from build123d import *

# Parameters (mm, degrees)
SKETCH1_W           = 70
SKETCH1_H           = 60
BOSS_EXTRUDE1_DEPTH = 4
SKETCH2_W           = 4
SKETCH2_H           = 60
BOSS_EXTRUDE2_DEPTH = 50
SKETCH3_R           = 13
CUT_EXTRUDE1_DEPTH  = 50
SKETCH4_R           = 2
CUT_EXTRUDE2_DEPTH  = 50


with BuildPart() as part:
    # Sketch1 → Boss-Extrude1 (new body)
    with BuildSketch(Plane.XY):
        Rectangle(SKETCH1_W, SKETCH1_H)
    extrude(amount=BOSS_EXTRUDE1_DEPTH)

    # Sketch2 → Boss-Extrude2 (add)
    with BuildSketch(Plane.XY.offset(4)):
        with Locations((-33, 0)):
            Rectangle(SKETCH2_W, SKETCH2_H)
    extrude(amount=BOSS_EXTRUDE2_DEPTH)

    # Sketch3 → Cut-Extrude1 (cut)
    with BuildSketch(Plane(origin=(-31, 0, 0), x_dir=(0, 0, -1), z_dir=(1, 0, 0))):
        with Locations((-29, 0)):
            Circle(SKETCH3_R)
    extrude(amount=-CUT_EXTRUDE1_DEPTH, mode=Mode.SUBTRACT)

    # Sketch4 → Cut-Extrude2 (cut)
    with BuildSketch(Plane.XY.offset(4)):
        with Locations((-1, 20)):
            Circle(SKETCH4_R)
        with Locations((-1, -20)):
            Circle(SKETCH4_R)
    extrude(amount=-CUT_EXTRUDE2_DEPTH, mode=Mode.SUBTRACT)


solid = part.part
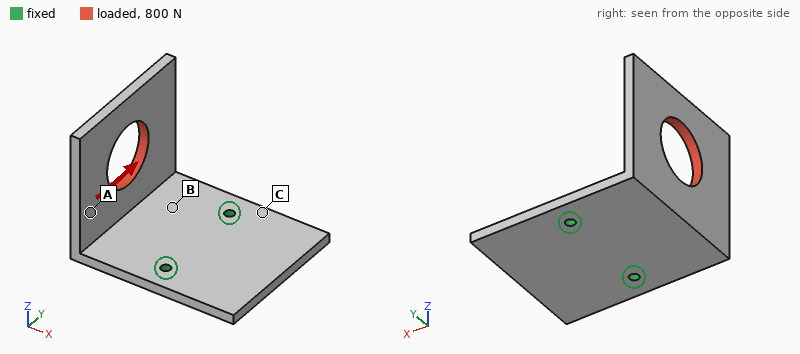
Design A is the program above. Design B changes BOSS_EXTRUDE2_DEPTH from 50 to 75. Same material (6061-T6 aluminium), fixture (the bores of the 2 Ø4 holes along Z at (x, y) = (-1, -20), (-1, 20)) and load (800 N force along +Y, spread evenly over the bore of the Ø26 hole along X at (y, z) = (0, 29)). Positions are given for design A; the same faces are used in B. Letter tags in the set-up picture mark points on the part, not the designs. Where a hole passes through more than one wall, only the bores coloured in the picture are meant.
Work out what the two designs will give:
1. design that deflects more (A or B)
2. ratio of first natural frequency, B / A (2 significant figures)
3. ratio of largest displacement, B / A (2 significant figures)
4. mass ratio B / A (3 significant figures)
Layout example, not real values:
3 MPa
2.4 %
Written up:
B
0.51
1.3
1.23
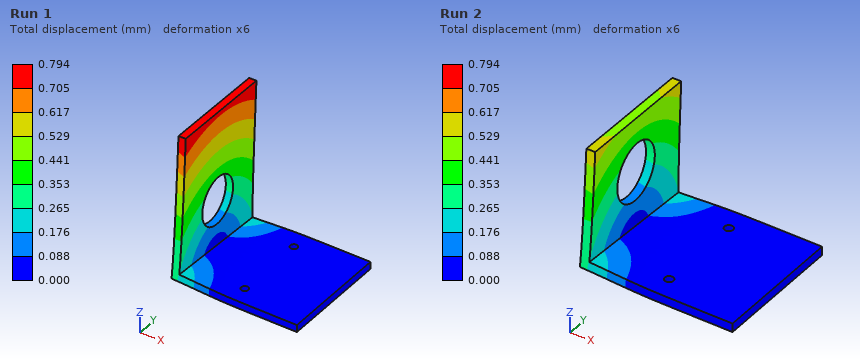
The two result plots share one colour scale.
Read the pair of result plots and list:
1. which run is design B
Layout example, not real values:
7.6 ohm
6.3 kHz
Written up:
Run 1
